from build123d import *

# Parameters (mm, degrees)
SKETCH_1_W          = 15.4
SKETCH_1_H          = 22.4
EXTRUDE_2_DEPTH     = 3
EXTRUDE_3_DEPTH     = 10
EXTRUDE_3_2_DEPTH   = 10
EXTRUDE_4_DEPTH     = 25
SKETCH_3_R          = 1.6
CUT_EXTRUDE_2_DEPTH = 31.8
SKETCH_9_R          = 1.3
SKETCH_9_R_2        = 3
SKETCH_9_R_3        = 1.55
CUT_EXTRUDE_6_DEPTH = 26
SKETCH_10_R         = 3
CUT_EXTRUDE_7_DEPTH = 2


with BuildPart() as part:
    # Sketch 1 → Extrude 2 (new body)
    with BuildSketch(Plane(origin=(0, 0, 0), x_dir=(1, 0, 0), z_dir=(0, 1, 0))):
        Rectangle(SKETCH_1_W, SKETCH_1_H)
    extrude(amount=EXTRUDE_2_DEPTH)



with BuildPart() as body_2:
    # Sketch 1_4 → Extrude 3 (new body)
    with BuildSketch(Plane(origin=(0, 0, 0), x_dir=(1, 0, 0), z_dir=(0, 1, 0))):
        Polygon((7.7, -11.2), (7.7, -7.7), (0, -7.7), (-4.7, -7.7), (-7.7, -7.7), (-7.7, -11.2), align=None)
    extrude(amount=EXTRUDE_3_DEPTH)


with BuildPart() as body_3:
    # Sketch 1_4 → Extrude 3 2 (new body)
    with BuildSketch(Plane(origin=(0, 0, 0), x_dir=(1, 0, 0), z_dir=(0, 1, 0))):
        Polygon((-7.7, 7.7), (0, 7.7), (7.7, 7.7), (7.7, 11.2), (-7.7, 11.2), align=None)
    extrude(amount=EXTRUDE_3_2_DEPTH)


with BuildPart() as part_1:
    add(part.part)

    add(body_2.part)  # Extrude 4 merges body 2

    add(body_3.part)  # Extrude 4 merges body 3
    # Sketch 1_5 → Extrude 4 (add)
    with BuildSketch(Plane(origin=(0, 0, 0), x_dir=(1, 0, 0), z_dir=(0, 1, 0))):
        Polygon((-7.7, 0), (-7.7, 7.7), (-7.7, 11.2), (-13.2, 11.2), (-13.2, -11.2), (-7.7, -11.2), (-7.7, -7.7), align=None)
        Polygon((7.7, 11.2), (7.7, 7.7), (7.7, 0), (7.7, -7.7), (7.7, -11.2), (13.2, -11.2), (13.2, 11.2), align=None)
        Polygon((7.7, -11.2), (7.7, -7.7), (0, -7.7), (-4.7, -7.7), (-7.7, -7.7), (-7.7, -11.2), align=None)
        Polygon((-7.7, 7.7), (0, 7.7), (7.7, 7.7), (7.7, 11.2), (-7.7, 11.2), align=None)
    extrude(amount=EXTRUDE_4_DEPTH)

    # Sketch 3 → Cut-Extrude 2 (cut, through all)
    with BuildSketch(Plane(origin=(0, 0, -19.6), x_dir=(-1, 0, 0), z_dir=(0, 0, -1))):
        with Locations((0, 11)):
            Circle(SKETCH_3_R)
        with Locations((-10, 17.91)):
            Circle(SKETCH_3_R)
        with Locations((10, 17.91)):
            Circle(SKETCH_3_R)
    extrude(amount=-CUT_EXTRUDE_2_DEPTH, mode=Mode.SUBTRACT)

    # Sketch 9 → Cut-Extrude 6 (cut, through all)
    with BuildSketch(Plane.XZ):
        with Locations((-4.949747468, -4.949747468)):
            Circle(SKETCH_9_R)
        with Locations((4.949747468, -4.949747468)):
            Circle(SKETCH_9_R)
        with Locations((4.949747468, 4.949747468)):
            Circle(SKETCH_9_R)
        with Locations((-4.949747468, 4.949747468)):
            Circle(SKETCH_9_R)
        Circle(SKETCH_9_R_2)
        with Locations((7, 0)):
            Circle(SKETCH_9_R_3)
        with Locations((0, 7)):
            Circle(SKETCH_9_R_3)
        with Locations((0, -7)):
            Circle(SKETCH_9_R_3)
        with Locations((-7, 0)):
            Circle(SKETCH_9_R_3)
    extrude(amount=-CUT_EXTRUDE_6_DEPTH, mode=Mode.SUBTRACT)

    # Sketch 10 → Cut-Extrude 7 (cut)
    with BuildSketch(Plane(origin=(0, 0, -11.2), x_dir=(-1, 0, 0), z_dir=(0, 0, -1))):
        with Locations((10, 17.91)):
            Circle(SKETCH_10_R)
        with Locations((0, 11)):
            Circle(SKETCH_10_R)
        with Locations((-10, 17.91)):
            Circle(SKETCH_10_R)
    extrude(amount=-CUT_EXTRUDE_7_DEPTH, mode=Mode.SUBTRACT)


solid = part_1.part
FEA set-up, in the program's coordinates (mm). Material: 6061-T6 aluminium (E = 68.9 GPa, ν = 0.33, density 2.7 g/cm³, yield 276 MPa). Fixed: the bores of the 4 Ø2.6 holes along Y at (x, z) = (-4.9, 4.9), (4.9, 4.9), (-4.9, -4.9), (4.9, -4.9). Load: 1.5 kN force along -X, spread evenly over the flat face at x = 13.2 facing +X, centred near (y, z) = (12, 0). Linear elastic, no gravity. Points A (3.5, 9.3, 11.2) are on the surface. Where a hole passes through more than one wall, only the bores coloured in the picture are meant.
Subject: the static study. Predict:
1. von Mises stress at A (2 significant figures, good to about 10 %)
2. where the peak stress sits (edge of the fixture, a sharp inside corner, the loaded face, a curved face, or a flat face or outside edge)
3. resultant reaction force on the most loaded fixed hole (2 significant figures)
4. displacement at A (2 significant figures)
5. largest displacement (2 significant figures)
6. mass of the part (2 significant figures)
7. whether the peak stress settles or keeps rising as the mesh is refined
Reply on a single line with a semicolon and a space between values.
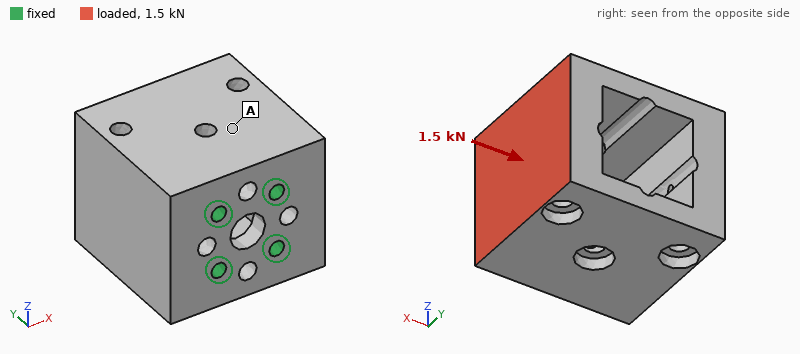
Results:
22 MPa; edge of the fixture; 760 N; 11 µm; 37 µm; 23 g; keeps rising
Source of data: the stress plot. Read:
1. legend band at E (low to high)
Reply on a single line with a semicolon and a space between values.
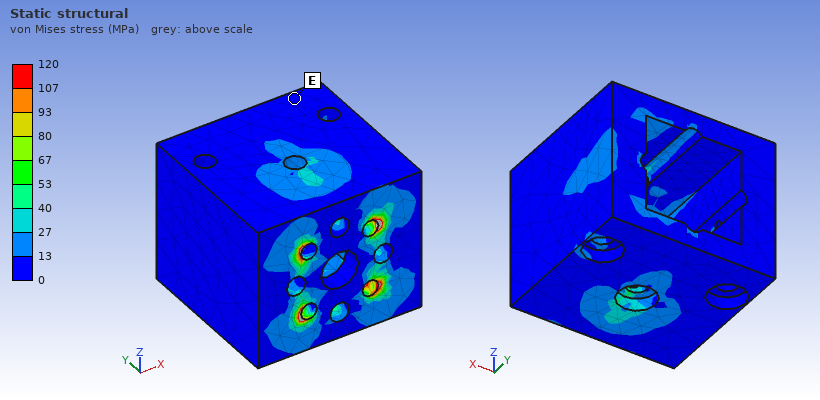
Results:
0 to 13 MPa
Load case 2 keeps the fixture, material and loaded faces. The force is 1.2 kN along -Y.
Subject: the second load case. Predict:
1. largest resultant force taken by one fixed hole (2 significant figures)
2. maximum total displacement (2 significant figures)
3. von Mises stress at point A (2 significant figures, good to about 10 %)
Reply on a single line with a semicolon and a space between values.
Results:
880 N; 28 µm; 13 MPa
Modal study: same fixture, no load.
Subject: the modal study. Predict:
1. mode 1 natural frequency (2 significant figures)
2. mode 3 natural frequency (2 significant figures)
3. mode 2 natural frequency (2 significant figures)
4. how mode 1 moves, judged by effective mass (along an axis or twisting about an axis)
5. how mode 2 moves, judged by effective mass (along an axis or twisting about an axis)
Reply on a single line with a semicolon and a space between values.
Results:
8300 Hz; 16 kHz; 9000 Hz; along X; along Z
